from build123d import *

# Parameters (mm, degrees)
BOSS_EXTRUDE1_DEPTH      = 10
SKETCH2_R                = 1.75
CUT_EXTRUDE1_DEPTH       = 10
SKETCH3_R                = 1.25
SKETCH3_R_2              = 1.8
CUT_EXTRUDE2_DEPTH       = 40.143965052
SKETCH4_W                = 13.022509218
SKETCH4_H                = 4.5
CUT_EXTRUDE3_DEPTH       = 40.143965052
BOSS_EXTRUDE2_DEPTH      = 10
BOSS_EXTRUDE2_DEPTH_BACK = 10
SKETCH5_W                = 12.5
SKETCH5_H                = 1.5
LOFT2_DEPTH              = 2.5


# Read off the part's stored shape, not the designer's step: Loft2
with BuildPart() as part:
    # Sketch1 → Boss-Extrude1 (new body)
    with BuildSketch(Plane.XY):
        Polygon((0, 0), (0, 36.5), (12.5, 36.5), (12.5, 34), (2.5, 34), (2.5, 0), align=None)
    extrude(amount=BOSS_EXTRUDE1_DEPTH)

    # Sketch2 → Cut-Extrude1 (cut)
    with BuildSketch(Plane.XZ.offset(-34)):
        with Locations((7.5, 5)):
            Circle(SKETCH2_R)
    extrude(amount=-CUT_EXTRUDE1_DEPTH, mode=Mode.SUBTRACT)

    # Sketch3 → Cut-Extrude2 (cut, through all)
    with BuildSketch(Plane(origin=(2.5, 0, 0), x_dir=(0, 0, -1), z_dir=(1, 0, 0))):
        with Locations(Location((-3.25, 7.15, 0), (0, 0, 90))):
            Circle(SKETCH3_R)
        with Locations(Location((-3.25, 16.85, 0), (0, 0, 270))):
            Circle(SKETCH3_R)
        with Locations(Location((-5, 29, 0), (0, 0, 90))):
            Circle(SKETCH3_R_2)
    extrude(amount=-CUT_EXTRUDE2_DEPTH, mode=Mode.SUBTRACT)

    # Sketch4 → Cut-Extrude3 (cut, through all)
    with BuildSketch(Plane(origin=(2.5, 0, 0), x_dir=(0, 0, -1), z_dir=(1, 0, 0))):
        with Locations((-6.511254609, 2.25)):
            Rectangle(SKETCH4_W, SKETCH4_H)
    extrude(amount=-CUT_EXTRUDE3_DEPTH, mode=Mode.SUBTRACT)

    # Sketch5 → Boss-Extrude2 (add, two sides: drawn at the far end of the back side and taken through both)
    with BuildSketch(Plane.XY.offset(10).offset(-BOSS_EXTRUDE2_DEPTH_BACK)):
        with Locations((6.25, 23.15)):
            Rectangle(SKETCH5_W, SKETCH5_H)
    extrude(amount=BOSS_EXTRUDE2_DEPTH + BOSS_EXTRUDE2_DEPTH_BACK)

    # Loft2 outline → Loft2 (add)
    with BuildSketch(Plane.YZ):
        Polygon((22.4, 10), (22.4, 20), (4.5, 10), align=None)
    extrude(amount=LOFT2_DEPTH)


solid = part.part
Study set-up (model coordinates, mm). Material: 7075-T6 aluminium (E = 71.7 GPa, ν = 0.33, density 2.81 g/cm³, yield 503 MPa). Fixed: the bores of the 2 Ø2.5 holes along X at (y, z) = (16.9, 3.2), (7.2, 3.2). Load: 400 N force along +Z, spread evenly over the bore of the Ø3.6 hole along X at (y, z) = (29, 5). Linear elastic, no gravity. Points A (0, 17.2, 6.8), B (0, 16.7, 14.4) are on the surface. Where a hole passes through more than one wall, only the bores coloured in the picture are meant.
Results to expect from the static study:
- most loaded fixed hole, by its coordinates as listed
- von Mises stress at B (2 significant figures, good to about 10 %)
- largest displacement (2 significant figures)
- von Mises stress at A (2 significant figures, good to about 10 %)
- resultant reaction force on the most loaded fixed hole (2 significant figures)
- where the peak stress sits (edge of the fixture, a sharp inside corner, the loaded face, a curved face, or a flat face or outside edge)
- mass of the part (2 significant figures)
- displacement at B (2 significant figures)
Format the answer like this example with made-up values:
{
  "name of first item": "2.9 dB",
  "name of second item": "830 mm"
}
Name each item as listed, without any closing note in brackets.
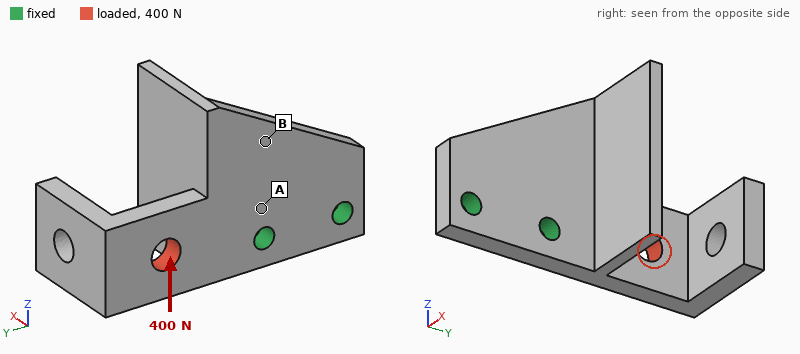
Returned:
{
  "most loaded fixed hole, by its coordinates as listed": "(16.9, 3.2)",
  "von Mises stress at B": "16 MPa",
  "largest displacement": "45 µm",
  "von Mises stress at A": "44 MPa",
  "resultant reaction force on the most loaded fixed hole": "770 N",
  "where the peak stress sits": "edge of the fixture",
  "mass of the part": "4.3 g",
  "displacement at B": "10.0 µm"
}
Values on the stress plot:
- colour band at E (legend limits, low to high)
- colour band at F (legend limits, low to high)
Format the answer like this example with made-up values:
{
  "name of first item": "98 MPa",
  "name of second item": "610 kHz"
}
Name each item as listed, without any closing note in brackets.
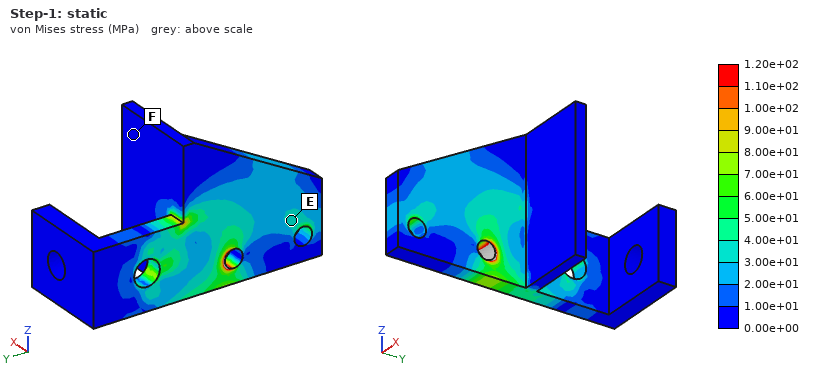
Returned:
{
  "colour band at E": "3.00e+01 to 4.00e+01 MPa",
  "colour band at F": "0.00e+00 to 1.00e+01 MPa"
}
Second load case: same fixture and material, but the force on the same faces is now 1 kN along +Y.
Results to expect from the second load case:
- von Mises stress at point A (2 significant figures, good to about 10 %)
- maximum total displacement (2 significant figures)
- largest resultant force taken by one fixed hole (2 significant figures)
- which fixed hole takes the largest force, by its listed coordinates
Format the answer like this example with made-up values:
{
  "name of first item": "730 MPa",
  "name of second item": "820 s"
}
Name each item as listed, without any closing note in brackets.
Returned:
{
  "von Mises stress at point A": "27 MPa",
  "maximum total displacement": "11 µm",
  "largest resultant force taken by one fixed hole": "850 N",
  "which fixed hole takes the largest force, by its listed coordinates": "(16.9, 3.2)"
}
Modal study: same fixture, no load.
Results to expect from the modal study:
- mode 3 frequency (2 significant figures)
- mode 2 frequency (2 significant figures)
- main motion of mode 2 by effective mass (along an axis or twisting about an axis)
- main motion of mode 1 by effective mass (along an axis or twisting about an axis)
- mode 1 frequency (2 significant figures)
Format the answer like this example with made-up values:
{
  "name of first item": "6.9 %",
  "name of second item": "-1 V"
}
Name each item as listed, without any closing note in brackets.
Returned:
{
  "mode 3 frequency": "8100 Hz",
  "mode 2 frequency": "5300 Hz",
  "main motion of mode 2 by effective mass": "along Z",
  "main motion of mode 1 by effective mass": "along X",
  "mode 1 frequency": "3100 Hz"
}
